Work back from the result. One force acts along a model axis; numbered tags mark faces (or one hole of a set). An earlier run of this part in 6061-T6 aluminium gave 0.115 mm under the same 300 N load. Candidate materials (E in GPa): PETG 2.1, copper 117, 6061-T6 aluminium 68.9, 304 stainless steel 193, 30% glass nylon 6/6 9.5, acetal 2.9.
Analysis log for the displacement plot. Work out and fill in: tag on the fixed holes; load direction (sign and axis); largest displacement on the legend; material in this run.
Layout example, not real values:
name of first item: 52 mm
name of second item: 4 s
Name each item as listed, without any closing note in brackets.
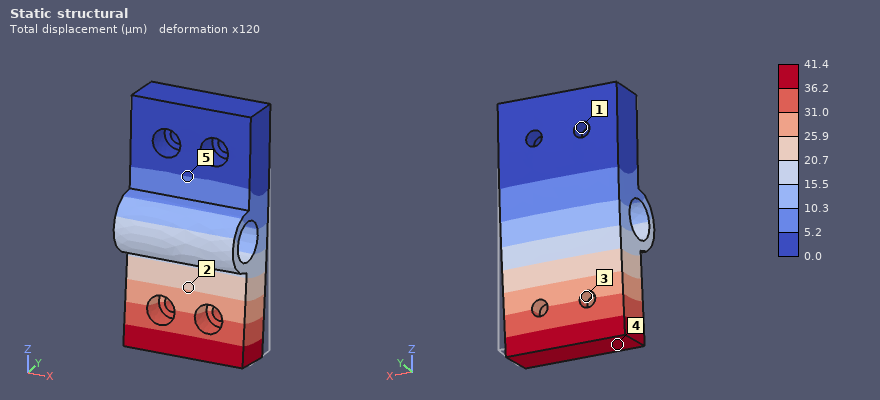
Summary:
tag on the fixed holes: 1
load direction: -Y
largest displacement on the legend: 41.4 µm
material in this run: 304 stainless steel
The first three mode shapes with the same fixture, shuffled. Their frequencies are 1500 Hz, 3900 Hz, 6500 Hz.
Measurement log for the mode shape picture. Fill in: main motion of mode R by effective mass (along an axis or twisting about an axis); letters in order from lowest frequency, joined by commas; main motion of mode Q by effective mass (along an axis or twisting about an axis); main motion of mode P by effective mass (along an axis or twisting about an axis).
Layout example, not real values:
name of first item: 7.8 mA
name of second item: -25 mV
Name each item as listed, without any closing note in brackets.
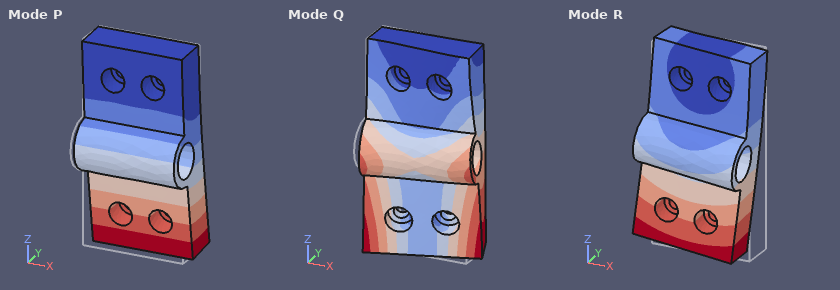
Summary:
main motion of mode R by effective mass: along X
letters in order from lowest frequency, joined by commas: P, R, Q
main motion of mode Q by effective mass: twisting about Z
main motion of mode P by effective mass: along Y
